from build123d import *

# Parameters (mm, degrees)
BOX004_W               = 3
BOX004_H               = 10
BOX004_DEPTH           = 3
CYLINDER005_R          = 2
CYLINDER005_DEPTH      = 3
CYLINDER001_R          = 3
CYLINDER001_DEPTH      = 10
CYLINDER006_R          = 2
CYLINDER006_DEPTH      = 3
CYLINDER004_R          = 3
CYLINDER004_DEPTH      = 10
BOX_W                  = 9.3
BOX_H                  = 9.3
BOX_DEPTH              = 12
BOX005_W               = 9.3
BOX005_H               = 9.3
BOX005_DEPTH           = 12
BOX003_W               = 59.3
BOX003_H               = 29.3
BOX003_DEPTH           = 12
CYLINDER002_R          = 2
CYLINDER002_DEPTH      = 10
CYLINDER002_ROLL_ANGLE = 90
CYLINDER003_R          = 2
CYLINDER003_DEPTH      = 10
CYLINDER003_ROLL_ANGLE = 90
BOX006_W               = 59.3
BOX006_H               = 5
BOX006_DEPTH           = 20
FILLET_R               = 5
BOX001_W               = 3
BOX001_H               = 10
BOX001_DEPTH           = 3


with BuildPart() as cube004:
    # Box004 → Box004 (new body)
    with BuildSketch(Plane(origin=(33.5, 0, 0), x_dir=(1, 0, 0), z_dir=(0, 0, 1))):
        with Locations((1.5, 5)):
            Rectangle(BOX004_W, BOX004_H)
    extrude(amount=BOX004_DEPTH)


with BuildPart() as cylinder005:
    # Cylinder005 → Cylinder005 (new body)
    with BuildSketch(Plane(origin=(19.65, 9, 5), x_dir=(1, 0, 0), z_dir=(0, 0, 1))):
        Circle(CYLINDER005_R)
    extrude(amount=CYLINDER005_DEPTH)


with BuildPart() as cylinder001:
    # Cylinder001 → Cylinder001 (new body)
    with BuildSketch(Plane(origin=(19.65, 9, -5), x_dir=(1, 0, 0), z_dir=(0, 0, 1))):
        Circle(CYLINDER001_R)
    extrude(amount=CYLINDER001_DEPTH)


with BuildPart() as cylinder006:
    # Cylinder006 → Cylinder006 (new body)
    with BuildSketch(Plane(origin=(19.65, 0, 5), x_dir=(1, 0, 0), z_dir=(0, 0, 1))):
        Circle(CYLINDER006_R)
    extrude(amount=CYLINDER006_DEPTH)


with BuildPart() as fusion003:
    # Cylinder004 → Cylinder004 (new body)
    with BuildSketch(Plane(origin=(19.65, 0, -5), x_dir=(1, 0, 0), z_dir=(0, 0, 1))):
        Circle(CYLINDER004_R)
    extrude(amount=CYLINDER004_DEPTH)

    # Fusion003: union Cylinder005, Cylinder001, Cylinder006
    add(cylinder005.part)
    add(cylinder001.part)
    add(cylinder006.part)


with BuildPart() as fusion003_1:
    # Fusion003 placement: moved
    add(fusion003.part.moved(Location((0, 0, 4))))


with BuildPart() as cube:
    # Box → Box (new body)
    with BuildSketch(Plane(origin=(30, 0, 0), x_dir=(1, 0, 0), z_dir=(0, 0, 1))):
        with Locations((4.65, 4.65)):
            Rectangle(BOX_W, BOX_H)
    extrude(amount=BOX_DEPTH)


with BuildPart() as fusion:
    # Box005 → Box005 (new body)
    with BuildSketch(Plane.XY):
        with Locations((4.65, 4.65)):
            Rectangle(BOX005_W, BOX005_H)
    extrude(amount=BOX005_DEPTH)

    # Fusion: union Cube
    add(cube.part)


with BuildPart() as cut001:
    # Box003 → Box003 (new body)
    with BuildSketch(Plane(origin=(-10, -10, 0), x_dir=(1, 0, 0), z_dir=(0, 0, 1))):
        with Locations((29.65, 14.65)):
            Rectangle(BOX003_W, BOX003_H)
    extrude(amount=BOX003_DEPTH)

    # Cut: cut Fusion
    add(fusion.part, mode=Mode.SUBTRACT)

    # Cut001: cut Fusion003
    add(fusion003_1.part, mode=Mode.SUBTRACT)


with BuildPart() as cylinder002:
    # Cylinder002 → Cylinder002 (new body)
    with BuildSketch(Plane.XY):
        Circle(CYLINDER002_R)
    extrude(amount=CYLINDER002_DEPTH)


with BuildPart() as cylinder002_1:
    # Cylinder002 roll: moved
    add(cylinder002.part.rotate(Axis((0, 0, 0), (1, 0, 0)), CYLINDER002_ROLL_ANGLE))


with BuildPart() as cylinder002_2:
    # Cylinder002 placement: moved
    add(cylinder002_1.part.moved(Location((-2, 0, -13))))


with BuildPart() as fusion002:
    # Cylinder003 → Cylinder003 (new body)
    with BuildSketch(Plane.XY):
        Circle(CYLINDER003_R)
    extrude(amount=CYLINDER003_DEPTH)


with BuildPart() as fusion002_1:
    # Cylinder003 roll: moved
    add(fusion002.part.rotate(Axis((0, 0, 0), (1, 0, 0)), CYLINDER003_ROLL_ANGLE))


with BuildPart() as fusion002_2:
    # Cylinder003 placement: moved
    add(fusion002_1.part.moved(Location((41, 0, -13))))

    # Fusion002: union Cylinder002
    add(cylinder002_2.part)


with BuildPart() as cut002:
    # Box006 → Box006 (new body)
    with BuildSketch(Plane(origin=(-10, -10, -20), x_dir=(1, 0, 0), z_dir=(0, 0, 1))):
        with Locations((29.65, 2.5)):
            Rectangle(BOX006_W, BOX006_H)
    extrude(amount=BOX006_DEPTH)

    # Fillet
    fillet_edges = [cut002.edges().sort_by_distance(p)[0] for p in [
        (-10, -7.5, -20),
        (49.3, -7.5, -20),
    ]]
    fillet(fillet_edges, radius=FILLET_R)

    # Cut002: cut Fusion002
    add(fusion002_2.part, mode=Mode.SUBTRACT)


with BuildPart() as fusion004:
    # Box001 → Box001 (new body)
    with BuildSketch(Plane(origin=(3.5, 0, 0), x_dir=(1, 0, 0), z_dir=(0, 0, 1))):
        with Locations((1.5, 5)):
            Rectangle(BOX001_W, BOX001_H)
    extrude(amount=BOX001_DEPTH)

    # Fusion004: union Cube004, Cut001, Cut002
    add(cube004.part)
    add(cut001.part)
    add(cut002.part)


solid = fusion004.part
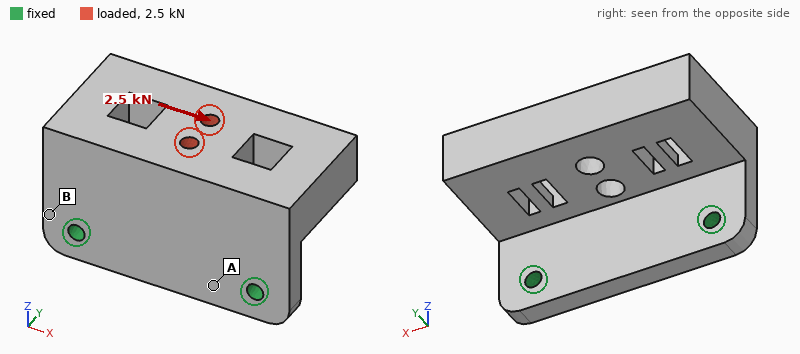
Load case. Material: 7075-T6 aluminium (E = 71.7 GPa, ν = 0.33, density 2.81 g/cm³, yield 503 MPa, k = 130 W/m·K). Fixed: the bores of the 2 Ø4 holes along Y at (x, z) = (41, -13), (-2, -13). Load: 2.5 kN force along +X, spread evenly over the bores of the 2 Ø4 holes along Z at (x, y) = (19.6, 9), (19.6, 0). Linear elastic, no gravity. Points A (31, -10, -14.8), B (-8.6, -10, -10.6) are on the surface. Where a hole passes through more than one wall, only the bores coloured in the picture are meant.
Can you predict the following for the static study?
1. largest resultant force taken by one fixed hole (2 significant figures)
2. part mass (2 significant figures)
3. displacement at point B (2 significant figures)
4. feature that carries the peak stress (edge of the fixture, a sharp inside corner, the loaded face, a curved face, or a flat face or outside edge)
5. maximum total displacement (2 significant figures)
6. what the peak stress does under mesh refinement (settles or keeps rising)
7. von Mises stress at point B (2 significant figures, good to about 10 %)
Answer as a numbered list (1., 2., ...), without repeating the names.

1. 1.9 kN
2. 68 g
3. 7.5 µm
4. edge of the fixture
5. 49 µm
6. keeps rising
7. 42 MPa
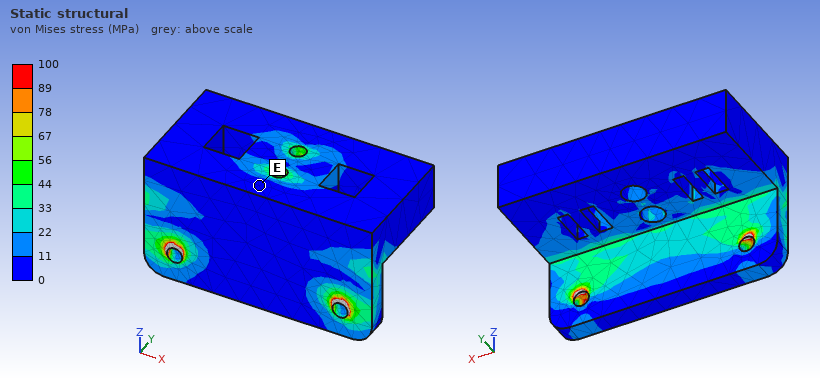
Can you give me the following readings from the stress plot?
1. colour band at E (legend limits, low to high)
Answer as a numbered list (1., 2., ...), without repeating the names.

1. 0 to 11 MPa
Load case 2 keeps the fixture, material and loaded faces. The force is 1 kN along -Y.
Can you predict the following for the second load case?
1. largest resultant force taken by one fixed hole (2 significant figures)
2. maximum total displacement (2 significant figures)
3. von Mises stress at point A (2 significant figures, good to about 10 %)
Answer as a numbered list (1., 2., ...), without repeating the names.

1. 500 N
2. 0.23 mm
3. 38 MPa
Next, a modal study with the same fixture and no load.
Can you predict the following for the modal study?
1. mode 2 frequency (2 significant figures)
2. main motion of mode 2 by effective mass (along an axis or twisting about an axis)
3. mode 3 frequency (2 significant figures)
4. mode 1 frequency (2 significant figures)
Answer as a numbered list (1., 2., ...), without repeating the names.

1. 4500 Hz
2. along X
3. 7100 Hz
4. 1700 Hz
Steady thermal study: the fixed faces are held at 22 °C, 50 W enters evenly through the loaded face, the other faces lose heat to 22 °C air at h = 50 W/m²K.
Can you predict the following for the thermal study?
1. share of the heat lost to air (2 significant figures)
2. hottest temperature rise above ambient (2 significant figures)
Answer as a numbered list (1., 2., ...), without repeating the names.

1. 20 %
2. 48 K
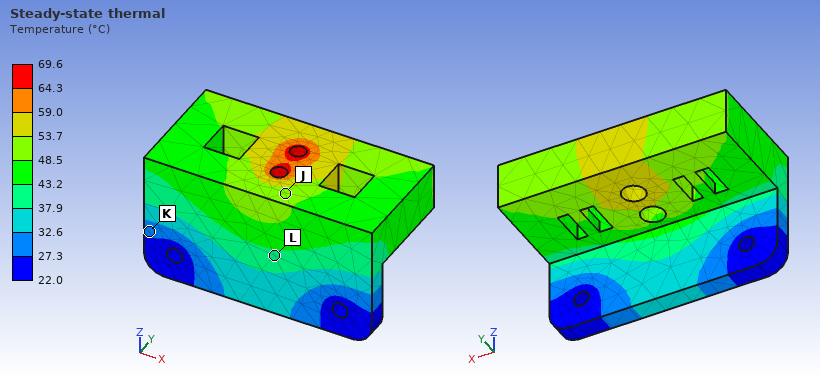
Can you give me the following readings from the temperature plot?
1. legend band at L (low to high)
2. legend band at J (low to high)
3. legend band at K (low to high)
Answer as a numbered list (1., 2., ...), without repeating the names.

1. 37.9 to 43.2 °C
2. 48.5 to 53.7 °C
3. 27.3 to 32.6 °C
